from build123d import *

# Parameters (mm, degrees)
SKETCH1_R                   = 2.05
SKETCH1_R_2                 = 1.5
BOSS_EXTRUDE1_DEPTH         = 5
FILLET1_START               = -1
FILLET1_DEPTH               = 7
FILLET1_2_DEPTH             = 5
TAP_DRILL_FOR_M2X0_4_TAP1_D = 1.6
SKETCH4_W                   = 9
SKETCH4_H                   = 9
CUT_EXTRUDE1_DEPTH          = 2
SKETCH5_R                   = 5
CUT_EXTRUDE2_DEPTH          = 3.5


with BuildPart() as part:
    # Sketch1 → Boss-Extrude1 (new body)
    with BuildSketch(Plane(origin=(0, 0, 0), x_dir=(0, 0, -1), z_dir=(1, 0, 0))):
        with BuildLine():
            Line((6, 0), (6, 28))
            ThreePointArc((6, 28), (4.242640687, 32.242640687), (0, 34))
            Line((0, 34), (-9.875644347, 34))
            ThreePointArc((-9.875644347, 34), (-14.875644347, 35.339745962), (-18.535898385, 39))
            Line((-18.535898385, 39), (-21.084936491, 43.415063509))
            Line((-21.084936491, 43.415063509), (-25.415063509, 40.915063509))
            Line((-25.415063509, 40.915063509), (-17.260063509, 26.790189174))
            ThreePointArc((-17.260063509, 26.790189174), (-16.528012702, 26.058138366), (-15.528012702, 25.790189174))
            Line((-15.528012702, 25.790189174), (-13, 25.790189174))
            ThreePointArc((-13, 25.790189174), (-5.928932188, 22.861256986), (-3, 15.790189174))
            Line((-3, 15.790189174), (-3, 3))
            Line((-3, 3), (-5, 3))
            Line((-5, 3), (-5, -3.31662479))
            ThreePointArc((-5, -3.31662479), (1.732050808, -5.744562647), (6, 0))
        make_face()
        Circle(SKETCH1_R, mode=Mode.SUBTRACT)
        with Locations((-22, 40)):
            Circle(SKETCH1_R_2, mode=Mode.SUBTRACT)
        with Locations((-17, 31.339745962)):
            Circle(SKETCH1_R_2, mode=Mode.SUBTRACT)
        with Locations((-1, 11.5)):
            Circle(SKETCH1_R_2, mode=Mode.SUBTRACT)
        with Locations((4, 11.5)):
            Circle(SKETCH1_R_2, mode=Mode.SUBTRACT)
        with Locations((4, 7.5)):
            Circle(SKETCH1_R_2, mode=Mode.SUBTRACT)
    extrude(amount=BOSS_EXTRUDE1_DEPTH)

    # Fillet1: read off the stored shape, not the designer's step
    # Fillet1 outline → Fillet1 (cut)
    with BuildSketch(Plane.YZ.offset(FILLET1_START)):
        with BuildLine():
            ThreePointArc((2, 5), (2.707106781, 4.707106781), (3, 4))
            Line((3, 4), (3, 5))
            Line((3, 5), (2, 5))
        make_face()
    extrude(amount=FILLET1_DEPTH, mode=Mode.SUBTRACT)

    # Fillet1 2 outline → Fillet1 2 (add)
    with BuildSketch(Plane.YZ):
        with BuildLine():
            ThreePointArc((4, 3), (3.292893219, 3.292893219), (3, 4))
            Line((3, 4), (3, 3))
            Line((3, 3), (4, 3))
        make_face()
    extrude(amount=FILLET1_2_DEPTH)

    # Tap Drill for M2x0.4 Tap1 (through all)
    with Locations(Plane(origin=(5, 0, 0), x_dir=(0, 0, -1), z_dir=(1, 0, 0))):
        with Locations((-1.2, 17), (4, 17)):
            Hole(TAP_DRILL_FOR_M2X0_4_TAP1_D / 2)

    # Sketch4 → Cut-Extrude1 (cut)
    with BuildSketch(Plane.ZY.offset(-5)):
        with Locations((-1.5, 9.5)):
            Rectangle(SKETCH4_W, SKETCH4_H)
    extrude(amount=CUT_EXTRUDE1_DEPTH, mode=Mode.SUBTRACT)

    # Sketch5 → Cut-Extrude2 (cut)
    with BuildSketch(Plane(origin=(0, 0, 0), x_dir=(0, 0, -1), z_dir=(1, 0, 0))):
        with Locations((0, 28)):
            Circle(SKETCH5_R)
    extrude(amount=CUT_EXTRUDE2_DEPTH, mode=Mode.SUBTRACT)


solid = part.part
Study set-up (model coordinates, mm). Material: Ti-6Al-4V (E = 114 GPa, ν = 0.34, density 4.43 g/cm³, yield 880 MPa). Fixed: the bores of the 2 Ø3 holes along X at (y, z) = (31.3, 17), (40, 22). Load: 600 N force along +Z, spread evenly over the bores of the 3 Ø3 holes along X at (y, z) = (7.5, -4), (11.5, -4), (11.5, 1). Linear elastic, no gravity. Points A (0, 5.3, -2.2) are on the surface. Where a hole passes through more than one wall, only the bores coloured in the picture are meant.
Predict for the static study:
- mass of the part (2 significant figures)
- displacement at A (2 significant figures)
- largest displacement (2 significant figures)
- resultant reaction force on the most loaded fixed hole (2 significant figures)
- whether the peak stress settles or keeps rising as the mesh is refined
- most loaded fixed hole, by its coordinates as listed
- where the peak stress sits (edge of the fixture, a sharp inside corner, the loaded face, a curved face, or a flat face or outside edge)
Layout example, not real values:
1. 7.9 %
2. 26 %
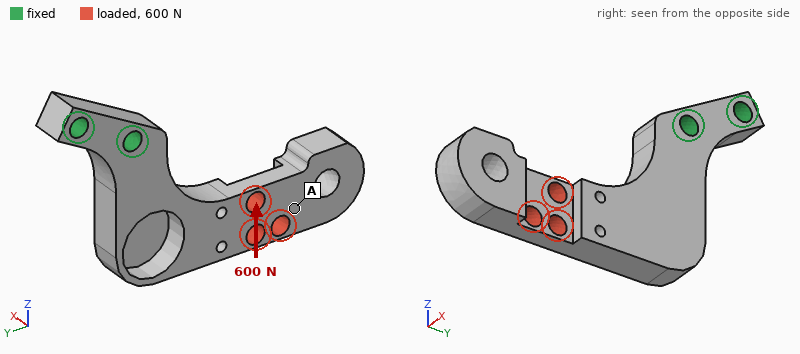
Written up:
1. 9.6 g
2. 0.27 mm
3. 0.38 mm
4. 1.2 kN
5. keeps rising
6. (31.3, 17)
7. edge of the fixture
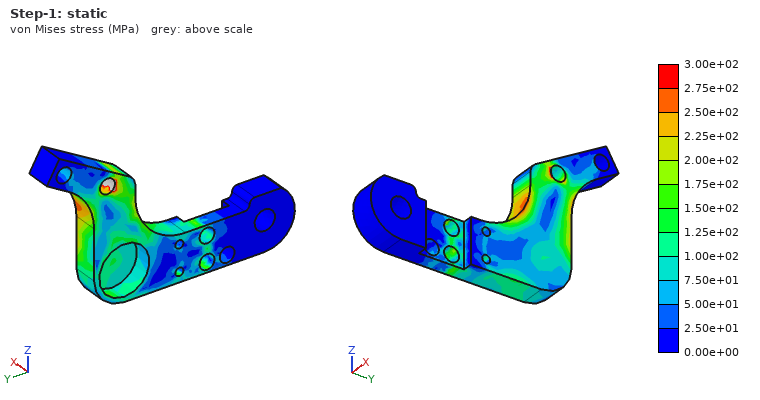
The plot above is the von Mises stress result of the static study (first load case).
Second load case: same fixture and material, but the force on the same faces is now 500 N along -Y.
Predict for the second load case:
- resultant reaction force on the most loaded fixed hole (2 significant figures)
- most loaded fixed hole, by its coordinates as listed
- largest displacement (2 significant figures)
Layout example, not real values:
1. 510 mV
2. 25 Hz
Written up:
1. 610 N
2. (31.3, 17)
3. 0.22 mm
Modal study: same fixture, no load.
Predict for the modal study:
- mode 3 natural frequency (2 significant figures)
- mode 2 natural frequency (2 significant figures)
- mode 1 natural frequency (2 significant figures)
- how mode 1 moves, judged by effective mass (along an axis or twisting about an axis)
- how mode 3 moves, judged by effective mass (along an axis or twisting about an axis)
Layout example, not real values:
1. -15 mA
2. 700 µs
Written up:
1. 5500 Hz
2. 3000 Hz
3. 1700 Hz
4. along X
5. along X
